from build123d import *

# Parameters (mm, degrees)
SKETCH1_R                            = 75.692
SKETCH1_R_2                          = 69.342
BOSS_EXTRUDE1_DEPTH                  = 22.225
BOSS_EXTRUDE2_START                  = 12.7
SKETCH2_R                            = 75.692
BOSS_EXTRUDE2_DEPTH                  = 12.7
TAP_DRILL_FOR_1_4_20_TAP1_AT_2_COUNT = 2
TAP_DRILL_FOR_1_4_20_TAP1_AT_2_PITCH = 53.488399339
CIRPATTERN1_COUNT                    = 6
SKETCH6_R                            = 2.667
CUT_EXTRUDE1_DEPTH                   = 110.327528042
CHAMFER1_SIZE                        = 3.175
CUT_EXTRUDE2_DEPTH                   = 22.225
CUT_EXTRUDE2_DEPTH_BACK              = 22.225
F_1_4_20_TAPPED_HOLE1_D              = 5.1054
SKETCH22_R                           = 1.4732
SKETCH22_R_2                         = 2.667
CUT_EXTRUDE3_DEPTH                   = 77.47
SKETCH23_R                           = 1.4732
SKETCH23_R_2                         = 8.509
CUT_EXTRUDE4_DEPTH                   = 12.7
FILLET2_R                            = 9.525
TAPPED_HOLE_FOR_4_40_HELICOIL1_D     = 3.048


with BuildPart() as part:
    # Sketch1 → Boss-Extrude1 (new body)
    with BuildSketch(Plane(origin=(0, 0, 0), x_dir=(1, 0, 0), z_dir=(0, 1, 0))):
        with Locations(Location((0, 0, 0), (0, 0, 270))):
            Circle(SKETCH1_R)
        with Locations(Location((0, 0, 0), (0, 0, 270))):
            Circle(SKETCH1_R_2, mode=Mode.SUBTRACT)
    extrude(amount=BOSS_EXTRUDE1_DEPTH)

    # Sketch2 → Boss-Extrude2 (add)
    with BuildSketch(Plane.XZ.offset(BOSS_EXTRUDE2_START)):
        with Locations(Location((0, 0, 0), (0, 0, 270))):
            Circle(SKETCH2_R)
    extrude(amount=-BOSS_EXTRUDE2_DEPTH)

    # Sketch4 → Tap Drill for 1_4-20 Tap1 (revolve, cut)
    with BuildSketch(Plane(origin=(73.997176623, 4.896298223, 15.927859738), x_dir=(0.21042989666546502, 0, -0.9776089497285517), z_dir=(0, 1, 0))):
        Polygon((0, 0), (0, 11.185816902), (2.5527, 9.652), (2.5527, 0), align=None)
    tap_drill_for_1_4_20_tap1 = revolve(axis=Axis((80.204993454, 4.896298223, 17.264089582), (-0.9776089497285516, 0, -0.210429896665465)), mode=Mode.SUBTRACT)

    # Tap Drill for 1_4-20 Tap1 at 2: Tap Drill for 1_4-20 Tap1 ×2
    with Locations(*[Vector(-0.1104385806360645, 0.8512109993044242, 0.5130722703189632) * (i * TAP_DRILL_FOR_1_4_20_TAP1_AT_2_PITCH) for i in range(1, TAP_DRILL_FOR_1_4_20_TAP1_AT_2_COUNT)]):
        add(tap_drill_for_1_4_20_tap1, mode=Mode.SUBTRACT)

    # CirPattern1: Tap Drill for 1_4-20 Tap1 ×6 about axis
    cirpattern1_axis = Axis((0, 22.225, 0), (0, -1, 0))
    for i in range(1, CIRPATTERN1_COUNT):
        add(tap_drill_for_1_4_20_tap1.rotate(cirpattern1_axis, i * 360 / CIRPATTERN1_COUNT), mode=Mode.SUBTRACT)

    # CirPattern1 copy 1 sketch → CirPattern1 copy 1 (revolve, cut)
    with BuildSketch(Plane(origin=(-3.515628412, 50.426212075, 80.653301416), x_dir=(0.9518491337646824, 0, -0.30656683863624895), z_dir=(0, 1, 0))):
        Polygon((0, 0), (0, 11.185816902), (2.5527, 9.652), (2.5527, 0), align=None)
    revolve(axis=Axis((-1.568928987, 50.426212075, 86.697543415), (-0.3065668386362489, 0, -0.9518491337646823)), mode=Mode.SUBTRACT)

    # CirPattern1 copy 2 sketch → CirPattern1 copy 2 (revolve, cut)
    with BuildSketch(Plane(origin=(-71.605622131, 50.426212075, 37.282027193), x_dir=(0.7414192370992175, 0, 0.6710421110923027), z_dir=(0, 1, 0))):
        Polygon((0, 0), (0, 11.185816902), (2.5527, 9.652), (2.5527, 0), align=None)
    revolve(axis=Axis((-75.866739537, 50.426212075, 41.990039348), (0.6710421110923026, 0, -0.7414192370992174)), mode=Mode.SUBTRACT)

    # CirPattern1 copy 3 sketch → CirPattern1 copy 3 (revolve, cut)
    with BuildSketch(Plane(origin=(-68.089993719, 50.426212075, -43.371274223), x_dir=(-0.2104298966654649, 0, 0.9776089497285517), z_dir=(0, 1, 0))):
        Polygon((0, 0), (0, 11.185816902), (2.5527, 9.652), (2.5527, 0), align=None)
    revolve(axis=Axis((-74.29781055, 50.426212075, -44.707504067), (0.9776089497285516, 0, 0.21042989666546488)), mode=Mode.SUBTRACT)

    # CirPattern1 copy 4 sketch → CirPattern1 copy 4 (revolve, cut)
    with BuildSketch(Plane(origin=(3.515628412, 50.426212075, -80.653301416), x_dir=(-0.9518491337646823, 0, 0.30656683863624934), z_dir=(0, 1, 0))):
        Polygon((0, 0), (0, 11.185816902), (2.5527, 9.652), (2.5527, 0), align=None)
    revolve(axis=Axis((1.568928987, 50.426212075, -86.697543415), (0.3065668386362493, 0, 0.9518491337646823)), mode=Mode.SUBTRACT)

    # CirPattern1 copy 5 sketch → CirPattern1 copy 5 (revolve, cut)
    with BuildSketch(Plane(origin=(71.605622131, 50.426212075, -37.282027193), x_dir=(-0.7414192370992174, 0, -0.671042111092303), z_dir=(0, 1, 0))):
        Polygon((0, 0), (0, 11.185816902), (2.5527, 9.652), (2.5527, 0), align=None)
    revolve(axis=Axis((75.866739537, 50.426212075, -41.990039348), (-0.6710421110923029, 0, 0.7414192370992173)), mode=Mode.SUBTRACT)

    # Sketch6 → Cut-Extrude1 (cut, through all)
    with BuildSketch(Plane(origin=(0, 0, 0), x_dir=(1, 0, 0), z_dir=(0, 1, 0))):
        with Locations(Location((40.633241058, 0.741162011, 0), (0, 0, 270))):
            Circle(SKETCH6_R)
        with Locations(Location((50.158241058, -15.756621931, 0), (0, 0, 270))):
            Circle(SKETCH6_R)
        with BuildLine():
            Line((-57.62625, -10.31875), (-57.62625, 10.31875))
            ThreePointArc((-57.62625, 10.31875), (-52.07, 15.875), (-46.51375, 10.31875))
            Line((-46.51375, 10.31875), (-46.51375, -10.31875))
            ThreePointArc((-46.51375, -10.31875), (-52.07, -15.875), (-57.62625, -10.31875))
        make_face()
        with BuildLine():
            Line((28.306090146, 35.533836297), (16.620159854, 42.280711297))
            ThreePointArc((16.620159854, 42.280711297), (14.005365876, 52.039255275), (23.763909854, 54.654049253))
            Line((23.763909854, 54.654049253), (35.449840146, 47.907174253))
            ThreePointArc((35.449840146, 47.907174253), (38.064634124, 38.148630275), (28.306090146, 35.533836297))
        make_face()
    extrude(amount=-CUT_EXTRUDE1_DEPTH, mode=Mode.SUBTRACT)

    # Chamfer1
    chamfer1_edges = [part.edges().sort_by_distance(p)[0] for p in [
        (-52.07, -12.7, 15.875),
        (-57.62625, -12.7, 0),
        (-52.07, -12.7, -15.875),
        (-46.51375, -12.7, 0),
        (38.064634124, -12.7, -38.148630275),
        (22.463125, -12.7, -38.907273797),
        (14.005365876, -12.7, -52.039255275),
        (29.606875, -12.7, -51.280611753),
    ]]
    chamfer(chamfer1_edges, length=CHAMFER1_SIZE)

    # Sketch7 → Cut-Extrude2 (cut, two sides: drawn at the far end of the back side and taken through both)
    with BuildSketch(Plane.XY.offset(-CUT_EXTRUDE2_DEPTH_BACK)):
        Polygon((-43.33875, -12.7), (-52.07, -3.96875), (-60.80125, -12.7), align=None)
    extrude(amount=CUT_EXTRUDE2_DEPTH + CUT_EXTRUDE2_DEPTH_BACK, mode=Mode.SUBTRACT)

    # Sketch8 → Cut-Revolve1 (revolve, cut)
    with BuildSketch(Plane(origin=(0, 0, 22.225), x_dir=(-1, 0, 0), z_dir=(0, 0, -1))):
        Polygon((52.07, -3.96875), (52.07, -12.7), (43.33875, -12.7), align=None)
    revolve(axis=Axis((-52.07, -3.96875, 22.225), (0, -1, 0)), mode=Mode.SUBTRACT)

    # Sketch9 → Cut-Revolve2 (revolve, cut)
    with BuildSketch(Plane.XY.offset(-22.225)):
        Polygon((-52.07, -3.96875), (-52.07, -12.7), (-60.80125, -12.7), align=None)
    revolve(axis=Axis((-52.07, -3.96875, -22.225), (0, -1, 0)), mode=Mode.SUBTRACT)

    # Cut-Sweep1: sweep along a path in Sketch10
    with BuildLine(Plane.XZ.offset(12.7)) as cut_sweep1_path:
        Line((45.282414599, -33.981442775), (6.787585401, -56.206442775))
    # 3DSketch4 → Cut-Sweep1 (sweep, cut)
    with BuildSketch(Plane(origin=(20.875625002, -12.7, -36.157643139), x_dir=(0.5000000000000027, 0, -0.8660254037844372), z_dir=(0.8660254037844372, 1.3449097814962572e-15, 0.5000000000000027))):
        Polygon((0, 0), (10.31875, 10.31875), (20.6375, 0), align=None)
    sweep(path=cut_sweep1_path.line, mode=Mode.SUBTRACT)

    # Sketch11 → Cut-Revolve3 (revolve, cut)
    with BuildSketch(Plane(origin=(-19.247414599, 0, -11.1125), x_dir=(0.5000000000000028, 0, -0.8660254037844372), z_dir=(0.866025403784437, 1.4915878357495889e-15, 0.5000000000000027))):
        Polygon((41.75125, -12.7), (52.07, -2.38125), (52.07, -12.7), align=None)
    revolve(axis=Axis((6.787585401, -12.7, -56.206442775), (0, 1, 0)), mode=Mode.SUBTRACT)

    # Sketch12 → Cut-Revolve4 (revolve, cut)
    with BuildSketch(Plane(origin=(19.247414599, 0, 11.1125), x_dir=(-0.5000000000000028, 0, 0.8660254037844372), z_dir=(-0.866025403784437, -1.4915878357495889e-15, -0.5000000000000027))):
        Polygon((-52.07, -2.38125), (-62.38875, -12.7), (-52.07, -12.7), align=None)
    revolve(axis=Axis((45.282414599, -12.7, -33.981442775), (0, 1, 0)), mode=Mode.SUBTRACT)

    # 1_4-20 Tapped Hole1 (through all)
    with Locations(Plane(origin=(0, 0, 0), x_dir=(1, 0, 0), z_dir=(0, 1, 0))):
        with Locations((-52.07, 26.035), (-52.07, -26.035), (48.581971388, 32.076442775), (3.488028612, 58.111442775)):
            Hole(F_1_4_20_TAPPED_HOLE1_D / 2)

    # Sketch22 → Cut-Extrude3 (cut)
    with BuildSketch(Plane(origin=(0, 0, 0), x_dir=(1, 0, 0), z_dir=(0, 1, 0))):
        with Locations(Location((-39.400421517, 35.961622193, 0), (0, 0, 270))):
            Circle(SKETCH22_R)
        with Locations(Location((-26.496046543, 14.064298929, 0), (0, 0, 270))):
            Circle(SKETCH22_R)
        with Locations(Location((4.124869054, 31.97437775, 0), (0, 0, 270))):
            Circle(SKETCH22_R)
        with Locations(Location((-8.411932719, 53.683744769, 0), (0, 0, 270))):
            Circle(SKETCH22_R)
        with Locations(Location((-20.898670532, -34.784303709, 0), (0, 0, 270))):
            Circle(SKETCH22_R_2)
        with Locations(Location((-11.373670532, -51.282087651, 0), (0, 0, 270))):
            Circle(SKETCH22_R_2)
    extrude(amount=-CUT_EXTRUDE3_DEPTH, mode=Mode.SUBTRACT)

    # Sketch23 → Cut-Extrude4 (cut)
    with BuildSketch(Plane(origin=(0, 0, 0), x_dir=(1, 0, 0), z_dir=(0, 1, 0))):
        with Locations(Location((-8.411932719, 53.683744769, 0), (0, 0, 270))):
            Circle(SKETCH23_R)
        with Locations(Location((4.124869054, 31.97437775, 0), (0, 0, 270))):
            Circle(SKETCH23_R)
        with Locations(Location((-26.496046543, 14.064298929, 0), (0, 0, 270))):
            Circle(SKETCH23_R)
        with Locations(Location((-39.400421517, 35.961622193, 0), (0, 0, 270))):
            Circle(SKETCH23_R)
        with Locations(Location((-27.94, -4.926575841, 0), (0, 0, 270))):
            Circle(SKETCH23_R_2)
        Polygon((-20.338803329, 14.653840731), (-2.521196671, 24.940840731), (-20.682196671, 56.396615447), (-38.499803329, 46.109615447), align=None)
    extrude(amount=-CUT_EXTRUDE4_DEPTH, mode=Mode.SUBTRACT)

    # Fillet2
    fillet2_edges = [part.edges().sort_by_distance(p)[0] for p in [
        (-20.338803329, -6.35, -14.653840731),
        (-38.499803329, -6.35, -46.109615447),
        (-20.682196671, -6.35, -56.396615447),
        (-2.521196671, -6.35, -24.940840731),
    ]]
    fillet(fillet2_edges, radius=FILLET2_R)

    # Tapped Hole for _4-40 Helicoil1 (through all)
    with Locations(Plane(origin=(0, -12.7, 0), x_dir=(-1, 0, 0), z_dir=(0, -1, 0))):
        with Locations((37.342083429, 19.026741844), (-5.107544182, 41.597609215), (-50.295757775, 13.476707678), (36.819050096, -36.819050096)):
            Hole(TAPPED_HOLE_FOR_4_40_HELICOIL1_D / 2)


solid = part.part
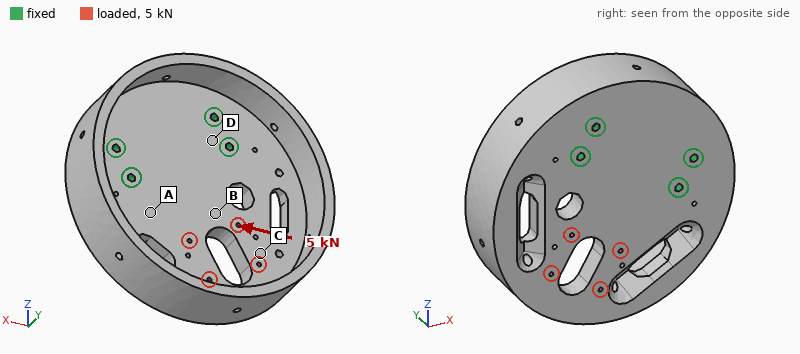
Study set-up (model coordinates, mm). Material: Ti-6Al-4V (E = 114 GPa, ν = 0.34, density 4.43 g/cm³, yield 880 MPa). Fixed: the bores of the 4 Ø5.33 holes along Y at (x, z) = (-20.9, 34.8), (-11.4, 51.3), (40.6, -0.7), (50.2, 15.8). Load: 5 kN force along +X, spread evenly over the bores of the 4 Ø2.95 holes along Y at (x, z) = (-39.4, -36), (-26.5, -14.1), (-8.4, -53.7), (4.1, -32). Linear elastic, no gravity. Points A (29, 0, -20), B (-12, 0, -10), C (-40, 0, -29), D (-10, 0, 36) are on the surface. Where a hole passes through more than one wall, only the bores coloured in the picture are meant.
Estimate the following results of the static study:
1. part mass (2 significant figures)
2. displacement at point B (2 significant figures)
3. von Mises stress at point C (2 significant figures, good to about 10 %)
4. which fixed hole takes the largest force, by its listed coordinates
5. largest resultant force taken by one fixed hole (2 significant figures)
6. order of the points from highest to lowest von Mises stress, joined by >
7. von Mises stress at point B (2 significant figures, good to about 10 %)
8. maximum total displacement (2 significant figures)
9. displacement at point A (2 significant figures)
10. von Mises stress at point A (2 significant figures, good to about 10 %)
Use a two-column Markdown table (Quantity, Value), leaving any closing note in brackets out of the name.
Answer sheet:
| Quantity | Value |
|---|---|
| part mass | 1.2 kg |
| displacement at point B | 4.9 µm |
| von Mises stress at point C | 6.1 MPa |
| which fixed hole takes the largest force, by its listed coordinates | (40.6, -0.7) |
| largest resultant force taken by one fixed hole | 4.0 kN |
| order of the points from highest to lowest von Mises stress, joined by > | B > A > C > D |
| von Mises stress at point B | 13 MPa |
| maximum total displacement | 12 µm |
| displacement at point A | 3.8 µm |
| von Mises stress at point A | 8.8 MPa |
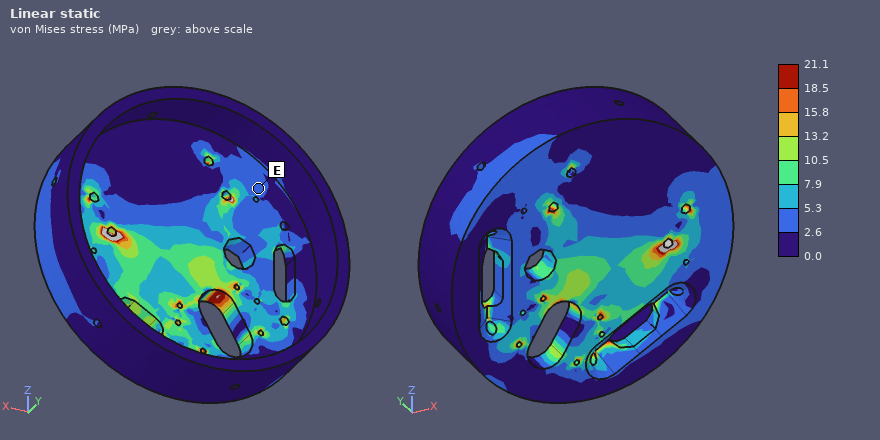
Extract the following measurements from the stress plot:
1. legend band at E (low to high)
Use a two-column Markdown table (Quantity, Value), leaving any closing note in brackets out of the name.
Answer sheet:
| Quantity | Value |
|---|---|
| legend band at E | 2.6 to 5.3 MPa |
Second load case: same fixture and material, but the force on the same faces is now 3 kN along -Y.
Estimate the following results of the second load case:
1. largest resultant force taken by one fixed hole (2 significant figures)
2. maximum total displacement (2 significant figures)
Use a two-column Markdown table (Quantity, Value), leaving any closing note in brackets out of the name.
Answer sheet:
| Quantity | Value |
|---|---|
| largest resultant force taken by one fixed hole | 3.7 kN |
| maximum total displacement | 0.14 mm |
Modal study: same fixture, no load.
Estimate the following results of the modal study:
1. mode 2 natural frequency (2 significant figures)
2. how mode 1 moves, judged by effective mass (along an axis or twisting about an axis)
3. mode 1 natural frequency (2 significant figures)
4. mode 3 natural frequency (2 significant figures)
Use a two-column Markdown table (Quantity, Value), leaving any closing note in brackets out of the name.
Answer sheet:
| Quantity | Value |
|---|---|
| mode 2 natural frequency | 2300 Hz |
| how mode 1 moves, judged by effective mass | along Y |
| mode 1 natural frequency | 1300 Hz |
| mode 3 natural frequency | 3500 Hz |
